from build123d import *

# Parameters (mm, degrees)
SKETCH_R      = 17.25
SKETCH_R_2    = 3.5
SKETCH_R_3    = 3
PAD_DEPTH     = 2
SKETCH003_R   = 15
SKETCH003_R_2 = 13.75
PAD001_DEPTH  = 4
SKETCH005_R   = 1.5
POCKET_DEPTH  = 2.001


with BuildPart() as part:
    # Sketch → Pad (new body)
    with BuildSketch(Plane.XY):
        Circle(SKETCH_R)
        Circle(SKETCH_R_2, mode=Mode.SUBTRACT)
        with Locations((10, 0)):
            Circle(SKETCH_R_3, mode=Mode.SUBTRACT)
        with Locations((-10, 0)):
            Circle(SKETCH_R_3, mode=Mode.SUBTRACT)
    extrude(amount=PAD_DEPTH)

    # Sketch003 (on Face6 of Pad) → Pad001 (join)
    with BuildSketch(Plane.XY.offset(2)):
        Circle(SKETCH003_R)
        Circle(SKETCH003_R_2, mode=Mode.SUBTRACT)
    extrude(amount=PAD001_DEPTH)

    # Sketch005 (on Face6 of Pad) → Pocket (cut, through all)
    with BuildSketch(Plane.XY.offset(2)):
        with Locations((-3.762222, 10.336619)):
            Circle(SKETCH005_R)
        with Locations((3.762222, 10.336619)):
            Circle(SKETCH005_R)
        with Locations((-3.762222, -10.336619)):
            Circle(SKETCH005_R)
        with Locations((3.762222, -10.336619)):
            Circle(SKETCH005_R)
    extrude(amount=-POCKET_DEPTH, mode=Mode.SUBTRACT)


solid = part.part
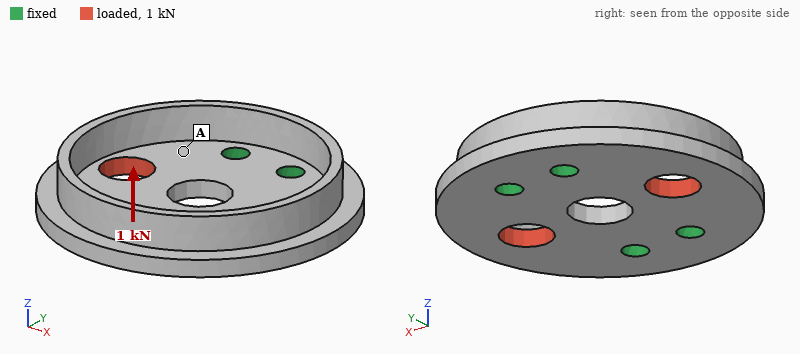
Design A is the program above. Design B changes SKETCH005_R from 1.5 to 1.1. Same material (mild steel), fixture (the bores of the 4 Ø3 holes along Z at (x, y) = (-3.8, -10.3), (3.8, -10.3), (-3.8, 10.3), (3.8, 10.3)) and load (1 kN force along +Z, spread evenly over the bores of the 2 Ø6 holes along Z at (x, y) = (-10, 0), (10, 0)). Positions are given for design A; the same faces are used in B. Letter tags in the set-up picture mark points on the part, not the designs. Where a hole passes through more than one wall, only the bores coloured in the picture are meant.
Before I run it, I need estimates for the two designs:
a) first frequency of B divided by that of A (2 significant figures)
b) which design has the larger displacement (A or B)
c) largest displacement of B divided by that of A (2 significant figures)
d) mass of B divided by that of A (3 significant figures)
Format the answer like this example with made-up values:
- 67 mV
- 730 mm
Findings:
- 0.93
- B
- 1.2
- 1.01
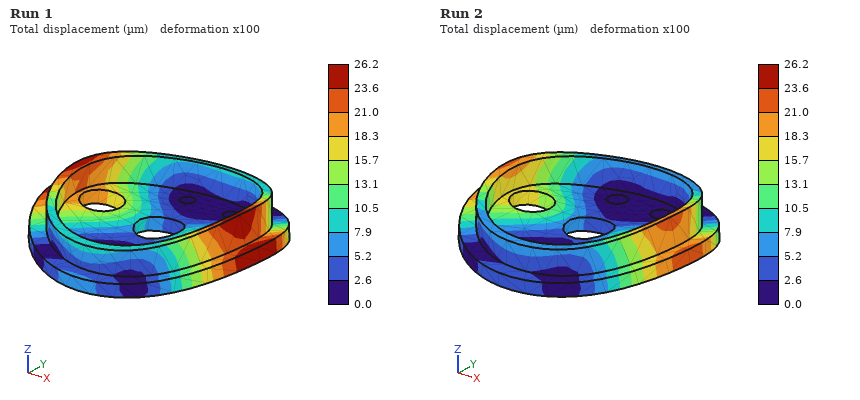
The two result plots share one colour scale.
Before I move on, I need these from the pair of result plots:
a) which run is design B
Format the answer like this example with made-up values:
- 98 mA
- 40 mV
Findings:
- Run 1
